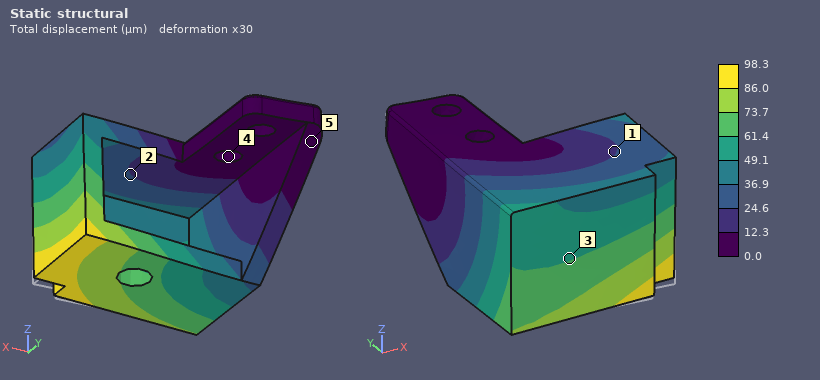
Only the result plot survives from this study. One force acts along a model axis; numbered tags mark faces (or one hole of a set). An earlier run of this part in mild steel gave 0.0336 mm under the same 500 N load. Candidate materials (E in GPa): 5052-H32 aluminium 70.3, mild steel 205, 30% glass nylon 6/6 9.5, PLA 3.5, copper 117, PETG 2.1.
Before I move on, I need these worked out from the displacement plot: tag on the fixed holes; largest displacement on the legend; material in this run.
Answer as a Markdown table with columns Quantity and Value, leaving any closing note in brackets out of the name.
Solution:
| Quantity | Value |
|---|---|
| tag on the fixed holes | 4 |
| largest displacement on the legend | 98.3 µm |
| material in this run | 5052-H32 aluminium |
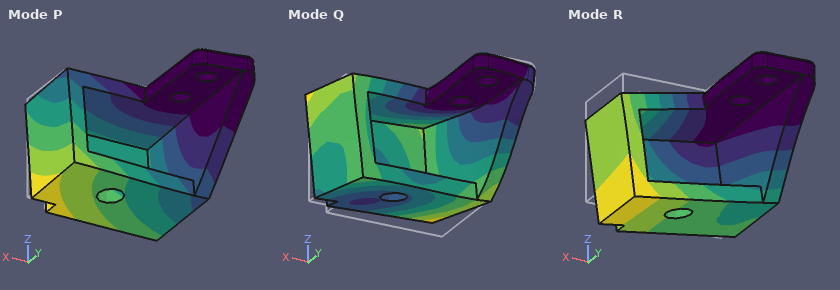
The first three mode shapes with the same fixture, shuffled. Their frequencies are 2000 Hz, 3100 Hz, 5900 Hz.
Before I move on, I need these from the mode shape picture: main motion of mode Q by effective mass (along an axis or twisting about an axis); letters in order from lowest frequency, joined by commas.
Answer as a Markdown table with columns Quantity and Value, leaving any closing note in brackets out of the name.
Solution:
| Quantity | Value |
|---|---|
| main motion of mode Q by effective mass | along Z |
| letters in order from lowest frequency, joined by commas | R, P, Q |
